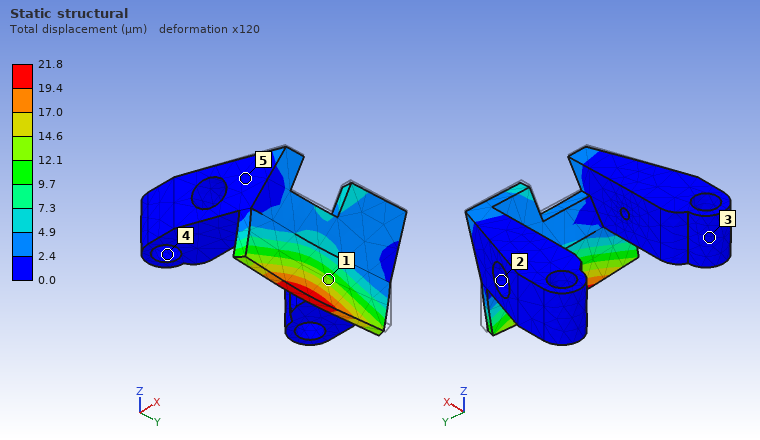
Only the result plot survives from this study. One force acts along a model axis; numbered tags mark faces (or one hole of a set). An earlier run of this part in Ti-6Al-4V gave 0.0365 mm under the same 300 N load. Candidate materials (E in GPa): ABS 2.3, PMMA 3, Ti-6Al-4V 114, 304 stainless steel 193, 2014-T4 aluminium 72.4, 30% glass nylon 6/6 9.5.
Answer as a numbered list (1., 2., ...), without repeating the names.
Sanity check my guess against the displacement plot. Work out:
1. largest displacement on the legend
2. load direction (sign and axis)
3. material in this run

1. 21.8 µm
2. -X
3. 304 stainless steel
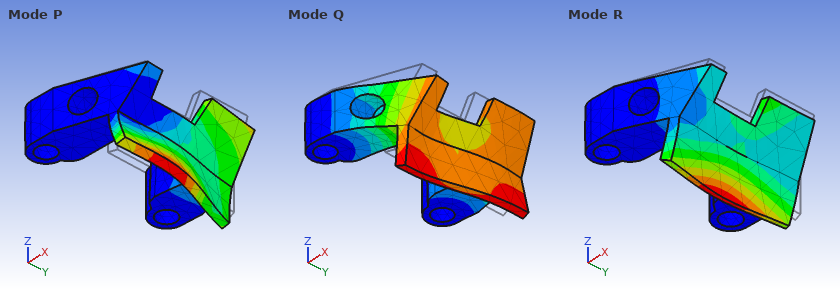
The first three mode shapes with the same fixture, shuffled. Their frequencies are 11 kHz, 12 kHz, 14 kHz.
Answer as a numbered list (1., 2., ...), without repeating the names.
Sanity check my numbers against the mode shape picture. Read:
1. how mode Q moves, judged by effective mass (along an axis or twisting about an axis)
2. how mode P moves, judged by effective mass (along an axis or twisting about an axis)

1. along Y
2. along Z
